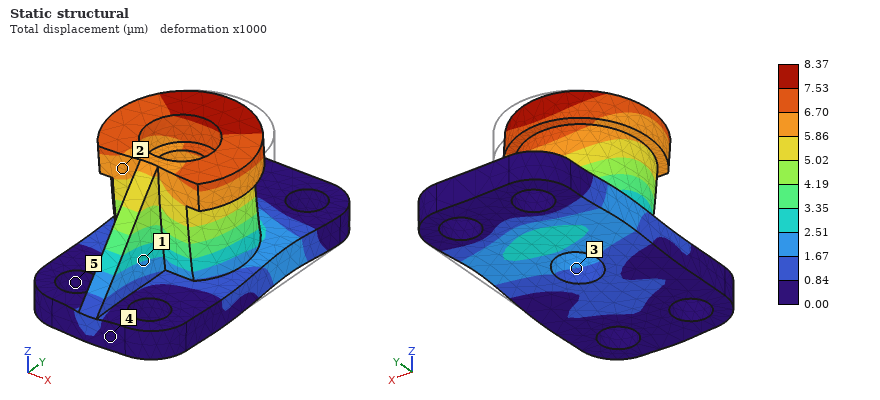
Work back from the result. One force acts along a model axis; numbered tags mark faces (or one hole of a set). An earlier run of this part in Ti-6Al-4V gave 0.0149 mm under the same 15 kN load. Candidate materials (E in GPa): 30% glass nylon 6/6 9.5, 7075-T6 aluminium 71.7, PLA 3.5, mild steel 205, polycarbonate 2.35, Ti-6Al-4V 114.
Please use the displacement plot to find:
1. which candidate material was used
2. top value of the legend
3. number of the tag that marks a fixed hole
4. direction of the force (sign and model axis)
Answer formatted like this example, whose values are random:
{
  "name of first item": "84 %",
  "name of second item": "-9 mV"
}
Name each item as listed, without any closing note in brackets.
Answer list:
{
  "which candidate material was used": "mild steel",
  "top value of the legend": "8.37 µm",
  "number of the tag that marks a fixed hole": "5",
  "direction of the force": "-Y"
}
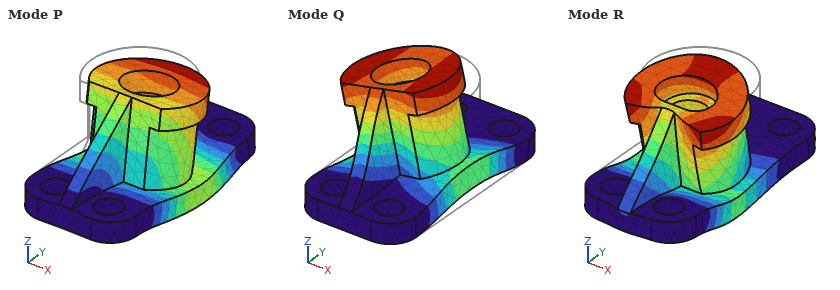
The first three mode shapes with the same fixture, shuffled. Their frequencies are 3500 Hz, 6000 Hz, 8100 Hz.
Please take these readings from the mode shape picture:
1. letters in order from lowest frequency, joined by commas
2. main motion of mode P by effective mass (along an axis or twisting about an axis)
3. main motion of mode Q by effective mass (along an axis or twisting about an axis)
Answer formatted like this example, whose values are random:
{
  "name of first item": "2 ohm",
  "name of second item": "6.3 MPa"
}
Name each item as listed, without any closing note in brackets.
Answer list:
{
  "letters in order from lowest frequency, joined by commas": "Q, P, R",
  "main motion of mode P by effective mass": "along Z",
  "main motion of mode Q by effective mass": "along X"
}
